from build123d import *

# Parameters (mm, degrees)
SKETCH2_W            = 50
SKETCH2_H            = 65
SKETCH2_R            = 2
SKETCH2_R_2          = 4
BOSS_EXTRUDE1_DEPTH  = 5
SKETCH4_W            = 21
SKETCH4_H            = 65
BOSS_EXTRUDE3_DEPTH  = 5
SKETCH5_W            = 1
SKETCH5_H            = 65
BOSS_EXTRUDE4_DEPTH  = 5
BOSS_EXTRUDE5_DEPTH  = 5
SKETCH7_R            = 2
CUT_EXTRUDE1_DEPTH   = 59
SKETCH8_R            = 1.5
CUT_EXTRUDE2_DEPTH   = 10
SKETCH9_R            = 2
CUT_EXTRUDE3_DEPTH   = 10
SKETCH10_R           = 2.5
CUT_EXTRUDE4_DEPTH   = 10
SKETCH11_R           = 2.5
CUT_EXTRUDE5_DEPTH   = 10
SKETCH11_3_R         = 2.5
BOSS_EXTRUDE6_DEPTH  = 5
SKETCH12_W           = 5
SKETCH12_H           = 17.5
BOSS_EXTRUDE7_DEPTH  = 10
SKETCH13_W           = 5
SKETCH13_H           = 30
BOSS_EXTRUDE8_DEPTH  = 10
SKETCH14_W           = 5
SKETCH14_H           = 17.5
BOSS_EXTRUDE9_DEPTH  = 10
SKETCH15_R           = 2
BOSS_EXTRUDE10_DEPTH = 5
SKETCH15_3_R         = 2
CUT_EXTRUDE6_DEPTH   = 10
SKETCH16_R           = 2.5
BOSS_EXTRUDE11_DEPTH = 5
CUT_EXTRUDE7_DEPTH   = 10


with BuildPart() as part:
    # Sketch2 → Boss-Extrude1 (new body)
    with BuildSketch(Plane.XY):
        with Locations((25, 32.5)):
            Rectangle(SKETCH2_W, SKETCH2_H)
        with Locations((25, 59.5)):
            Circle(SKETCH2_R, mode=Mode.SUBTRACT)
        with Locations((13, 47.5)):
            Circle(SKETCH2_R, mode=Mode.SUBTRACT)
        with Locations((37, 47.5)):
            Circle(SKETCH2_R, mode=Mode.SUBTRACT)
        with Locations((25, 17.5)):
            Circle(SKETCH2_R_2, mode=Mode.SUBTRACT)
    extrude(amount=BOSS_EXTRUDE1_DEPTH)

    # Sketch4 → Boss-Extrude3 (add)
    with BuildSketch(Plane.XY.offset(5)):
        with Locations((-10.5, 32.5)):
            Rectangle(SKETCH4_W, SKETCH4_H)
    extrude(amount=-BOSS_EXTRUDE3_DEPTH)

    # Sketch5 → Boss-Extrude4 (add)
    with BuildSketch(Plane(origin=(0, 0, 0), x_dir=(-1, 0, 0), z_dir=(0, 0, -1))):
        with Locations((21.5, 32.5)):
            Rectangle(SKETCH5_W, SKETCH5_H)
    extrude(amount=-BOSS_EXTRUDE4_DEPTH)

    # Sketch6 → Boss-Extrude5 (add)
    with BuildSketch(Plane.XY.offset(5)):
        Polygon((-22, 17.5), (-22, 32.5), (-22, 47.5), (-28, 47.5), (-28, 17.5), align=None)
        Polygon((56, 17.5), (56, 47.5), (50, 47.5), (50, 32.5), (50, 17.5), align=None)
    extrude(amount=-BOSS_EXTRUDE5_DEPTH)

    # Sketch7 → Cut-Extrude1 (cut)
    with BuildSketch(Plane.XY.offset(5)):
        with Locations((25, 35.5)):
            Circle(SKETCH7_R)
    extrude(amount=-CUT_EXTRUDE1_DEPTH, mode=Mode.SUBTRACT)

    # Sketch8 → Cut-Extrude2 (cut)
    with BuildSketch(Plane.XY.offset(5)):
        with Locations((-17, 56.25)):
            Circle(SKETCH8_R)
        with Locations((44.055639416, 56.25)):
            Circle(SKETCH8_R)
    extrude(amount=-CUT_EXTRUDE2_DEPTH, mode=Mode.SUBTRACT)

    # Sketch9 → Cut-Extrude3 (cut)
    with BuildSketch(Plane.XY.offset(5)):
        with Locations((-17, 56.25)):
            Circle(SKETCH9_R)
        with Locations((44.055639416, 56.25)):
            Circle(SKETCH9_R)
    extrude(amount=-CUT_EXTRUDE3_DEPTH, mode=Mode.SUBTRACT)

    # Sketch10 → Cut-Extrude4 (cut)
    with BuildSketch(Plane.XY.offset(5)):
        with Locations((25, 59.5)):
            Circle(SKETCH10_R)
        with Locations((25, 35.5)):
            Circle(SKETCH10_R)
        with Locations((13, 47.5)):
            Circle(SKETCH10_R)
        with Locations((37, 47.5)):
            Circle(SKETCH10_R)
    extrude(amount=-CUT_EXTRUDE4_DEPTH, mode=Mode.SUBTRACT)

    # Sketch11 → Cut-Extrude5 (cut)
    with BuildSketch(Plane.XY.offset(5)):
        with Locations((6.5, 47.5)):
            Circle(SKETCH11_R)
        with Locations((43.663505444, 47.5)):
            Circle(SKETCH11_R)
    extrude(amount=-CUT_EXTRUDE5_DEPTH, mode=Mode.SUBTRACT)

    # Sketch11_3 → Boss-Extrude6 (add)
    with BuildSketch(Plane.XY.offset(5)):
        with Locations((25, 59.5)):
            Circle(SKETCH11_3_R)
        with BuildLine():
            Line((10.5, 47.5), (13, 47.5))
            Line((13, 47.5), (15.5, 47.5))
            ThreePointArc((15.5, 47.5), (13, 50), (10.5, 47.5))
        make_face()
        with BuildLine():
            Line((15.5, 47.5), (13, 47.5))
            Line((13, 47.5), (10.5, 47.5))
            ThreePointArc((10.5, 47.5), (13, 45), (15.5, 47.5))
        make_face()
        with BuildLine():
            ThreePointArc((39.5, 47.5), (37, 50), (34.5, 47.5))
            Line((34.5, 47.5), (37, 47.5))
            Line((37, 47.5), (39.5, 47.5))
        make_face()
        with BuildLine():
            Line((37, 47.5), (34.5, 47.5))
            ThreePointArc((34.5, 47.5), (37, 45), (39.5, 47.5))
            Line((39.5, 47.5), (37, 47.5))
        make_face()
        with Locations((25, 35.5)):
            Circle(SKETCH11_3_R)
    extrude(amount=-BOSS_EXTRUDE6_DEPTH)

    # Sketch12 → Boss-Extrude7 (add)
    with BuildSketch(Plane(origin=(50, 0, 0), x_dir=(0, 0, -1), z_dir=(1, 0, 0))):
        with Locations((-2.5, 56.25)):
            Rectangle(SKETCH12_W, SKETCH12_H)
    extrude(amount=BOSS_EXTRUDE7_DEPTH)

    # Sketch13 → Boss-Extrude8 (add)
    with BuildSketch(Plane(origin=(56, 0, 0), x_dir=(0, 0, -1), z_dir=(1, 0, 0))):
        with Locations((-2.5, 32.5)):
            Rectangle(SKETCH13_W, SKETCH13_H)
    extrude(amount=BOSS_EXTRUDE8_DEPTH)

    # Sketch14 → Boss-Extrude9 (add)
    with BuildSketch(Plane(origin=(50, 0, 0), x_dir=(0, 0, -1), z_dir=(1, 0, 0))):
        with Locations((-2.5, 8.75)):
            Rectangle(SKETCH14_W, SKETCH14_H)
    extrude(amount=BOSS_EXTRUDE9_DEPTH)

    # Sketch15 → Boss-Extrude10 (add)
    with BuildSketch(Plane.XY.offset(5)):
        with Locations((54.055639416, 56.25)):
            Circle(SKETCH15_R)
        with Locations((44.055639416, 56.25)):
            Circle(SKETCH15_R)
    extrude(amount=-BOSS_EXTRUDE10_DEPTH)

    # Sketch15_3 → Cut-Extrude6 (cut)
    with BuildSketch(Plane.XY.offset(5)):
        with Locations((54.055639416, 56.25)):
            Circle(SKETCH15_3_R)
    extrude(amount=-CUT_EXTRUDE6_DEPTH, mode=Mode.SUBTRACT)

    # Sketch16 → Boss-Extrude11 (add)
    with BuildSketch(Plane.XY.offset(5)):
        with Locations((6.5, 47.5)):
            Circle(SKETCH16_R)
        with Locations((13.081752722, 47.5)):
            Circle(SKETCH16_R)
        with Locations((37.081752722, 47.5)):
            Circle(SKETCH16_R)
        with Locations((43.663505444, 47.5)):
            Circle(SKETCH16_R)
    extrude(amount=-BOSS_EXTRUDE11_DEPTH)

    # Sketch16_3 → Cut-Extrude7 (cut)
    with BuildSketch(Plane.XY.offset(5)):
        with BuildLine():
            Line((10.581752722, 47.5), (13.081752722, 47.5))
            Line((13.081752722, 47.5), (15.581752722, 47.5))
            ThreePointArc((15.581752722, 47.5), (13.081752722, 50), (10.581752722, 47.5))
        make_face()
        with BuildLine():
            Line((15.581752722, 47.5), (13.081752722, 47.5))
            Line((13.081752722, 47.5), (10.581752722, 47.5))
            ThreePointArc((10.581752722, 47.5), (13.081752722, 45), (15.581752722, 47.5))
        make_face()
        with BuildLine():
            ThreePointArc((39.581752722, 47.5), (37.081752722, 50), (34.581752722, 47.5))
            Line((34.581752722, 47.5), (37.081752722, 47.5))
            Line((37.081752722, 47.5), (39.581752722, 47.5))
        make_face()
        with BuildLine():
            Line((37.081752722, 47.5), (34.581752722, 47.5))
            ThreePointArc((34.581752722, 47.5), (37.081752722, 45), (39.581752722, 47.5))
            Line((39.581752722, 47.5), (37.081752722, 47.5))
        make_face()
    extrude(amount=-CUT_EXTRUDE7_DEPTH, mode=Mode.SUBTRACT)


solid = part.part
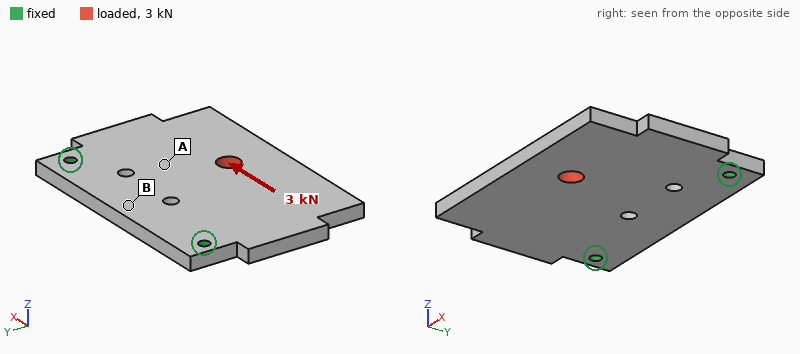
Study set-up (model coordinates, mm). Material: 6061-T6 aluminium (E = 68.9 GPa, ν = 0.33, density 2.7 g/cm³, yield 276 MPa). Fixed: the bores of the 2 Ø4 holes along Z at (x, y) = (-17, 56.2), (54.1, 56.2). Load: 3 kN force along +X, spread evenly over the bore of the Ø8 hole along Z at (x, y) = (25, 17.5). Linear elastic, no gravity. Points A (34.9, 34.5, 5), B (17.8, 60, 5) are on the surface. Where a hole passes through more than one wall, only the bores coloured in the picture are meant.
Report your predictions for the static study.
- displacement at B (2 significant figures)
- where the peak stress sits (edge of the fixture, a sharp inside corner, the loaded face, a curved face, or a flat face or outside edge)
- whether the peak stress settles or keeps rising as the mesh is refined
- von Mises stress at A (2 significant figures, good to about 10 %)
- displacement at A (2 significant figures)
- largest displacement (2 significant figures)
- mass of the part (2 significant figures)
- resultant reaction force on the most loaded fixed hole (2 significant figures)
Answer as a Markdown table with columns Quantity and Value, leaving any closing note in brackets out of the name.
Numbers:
| Quantity | Value |
|---|---|
| displacement at B | 3.8 µm |
| where the peak stress sits | edge of the fixture |
| whether the peak stress settles or keeps rising as the mesh is refined | keeps rising |
| von Mises stress at A | 17 MPa |
| displacement at A | 12 µm |
| largest displacement | 25 µm |
| mass of the part | 75 g |
| resultant reaction force on the most loaded fixed hole | 2.2 kN |
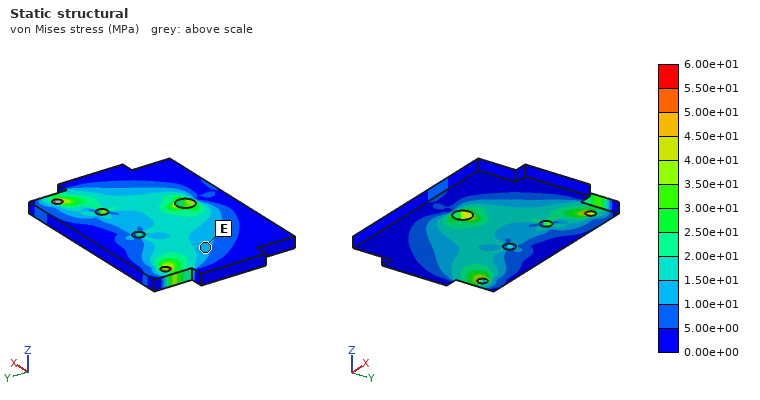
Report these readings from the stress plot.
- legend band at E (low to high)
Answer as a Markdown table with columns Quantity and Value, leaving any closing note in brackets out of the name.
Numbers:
| Quantity | Value |
|---|---|
| legend band at E | 1.00e+01 to 1.50e+01 MPa |
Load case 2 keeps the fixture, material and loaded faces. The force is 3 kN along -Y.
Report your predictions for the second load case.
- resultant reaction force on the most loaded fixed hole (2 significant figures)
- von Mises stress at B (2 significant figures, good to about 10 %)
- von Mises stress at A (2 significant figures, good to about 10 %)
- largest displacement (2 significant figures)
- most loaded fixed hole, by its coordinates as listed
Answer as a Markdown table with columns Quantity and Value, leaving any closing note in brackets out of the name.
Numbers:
| Quantity | Value |
|---|---|
| resultant reaction force on the most loaded fixed hole | 1.9 kN |
| von Mises stress at B | 6.4 MPa |
| von Mises stress at A | 15 MPa |
| largest displacement | 16 µm |
| most loaded fixed hole, by its coordinates as listed | (54.1, 56.2) |
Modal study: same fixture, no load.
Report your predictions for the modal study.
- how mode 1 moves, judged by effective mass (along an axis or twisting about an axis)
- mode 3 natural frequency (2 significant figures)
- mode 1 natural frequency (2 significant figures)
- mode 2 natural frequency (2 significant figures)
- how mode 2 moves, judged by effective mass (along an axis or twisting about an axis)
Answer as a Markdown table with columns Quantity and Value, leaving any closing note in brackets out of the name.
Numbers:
| Quantity | Value |
|---|---|
| how mode 1 moves, judged by effective mass | along Z |
| mode 3 natural frequency | 4200 Hz |
| mode 1 natural frequency | 980 Hz |
| mode 2 natural frequency | 2300 Hz |
| how mode 2 moves, judged by effective mass | twisting about Y |
